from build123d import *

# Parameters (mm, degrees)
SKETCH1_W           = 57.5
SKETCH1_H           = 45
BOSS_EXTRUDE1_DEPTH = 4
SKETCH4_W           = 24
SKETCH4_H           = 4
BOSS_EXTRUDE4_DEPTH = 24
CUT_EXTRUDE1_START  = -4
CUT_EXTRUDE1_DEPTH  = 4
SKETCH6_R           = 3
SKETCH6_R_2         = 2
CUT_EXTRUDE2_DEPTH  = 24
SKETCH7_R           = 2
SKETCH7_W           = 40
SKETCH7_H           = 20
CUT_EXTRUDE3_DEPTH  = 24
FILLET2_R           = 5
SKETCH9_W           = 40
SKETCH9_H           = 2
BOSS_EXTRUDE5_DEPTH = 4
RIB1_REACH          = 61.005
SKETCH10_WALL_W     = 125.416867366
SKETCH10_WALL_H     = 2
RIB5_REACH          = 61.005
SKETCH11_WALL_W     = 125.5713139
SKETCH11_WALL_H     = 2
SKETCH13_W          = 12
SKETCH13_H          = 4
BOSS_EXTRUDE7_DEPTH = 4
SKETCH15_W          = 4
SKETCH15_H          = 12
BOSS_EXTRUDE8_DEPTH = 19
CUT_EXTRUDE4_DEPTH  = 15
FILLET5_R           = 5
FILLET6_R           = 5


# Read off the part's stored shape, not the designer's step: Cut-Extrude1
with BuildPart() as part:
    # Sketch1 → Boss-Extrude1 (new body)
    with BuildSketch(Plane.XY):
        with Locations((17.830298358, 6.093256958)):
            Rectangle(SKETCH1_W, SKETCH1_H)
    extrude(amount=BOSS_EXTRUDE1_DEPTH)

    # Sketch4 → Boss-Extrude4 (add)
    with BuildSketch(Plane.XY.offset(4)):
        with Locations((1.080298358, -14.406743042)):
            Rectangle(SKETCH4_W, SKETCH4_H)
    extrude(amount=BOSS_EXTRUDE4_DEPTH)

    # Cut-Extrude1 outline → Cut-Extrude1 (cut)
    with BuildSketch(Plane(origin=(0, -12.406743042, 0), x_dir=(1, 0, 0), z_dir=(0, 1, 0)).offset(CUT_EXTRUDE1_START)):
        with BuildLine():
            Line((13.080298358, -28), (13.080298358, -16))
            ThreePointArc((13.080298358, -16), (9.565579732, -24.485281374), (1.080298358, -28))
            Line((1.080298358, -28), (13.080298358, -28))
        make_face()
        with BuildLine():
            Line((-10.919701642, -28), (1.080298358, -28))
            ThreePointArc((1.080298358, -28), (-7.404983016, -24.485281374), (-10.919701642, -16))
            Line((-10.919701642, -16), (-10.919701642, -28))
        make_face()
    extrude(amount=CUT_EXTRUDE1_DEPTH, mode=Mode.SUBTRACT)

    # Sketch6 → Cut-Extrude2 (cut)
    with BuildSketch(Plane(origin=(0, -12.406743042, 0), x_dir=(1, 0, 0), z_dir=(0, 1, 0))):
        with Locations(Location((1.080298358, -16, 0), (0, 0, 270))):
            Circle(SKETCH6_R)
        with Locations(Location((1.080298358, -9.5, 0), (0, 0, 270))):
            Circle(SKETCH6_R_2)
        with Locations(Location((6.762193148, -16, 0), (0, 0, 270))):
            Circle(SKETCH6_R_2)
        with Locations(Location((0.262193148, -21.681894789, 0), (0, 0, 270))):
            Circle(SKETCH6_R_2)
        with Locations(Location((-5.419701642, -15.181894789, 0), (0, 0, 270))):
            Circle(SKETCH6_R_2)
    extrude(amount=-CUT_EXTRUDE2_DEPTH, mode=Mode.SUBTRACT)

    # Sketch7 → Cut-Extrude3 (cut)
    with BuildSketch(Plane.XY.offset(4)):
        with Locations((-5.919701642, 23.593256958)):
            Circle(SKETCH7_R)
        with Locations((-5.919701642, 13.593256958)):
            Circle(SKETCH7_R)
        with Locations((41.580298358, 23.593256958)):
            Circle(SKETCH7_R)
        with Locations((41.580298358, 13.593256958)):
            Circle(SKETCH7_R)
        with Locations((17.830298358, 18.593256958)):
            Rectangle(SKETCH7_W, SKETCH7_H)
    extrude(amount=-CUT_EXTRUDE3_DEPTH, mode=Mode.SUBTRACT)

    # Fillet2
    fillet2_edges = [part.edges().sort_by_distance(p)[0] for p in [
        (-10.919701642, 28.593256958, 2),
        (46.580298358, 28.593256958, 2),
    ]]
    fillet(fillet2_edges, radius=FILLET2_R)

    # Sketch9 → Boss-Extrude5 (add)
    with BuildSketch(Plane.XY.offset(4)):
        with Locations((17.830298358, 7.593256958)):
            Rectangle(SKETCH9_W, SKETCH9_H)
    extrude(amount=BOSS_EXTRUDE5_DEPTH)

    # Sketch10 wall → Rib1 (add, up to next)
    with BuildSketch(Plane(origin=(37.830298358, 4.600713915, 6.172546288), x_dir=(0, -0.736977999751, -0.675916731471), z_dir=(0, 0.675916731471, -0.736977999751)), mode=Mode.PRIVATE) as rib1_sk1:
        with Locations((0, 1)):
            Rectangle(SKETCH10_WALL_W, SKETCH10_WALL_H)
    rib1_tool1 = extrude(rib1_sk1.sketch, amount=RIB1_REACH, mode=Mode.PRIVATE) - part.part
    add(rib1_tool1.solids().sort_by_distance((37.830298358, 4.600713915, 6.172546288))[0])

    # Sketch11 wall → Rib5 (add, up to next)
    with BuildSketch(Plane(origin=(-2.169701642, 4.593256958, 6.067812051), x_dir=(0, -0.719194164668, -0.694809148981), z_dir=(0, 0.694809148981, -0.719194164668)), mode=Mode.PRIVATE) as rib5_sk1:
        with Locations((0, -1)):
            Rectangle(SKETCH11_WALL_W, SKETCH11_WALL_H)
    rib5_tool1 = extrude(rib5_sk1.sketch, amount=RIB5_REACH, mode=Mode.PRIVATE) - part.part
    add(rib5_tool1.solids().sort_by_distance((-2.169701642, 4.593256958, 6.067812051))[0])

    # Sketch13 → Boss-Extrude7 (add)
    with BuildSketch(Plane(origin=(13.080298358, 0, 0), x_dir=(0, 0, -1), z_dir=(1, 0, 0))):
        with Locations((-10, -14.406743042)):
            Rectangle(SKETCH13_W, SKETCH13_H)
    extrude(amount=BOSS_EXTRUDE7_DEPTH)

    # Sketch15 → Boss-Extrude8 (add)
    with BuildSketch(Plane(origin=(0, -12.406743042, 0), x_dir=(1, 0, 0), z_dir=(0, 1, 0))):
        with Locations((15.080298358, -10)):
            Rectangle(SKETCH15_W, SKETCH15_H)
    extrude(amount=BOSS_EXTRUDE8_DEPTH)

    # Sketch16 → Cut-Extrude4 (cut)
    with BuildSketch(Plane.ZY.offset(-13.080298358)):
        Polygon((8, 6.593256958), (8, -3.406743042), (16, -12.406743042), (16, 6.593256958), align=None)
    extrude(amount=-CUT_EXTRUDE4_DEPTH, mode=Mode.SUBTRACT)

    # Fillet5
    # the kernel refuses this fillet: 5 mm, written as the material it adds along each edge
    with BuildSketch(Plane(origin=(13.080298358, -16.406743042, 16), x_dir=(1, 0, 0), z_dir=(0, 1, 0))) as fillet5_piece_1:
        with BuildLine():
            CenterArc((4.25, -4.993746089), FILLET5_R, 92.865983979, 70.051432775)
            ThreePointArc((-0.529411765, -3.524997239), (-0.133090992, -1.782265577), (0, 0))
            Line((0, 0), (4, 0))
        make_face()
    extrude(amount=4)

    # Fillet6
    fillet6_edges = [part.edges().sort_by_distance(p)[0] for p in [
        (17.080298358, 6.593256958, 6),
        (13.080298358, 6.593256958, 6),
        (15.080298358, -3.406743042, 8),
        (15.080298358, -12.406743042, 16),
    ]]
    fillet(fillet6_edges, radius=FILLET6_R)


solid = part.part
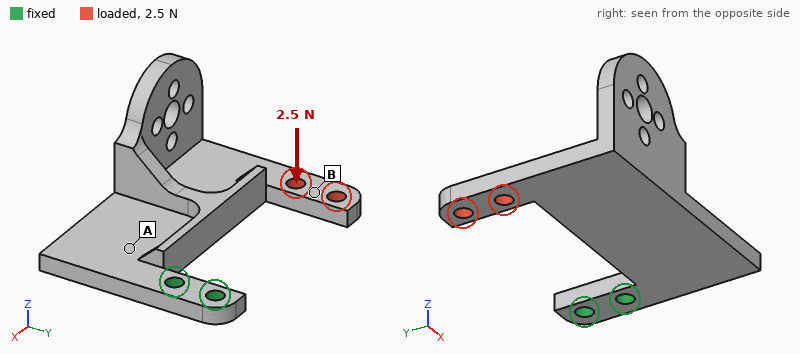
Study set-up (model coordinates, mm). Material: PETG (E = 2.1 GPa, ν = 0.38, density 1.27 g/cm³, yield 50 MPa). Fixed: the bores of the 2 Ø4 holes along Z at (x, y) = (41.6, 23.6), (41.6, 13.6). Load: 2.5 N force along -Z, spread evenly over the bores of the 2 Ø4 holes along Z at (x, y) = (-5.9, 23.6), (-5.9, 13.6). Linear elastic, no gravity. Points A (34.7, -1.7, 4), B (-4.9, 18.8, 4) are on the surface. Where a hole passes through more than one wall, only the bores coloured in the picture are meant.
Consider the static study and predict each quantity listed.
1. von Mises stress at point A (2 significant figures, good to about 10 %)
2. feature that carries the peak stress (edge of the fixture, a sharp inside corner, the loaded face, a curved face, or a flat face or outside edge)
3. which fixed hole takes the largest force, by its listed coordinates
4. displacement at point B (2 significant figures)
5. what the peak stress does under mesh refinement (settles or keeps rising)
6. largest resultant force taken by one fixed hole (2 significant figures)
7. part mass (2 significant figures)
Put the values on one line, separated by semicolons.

1.2 MPa; edge of the fixture; (41.6, 13.6); 0.72 mm; keeps rising; 2.0 N; 12 g
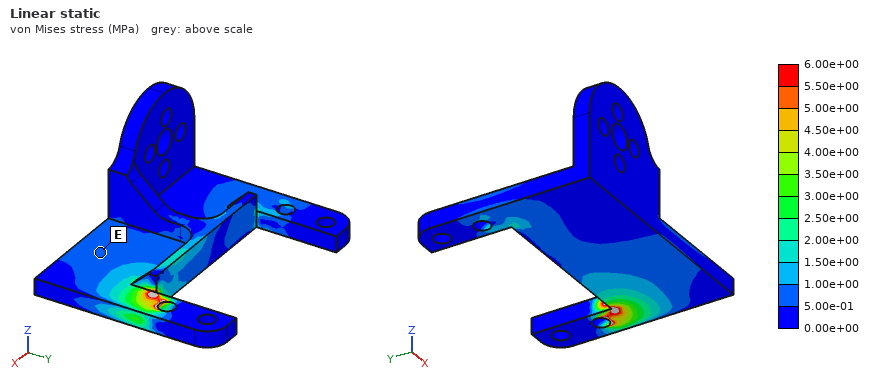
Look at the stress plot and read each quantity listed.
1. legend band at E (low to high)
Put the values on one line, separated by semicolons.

5.00e-01 to 1.00e+00 MPa
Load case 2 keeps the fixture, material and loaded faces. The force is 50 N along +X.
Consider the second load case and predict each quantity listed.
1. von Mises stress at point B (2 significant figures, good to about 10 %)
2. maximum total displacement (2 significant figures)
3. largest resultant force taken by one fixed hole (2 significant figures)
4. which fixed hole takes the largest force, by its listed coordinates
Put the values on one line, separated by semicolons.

2.6 MPa; 0.93 mm; 42 N; (41.6, 13.6)
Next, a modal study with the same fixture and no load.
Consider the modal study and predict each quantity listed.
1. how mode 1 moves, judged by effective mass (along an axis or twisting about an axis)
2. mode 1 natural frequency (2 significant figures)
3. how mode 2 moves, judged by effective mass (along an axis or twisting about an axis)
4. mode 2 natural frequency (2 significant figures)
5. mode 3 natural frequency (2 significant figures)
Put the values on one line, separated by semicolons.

along Z; 130 Hz; along Y; 240 Hz; 340 Hz
